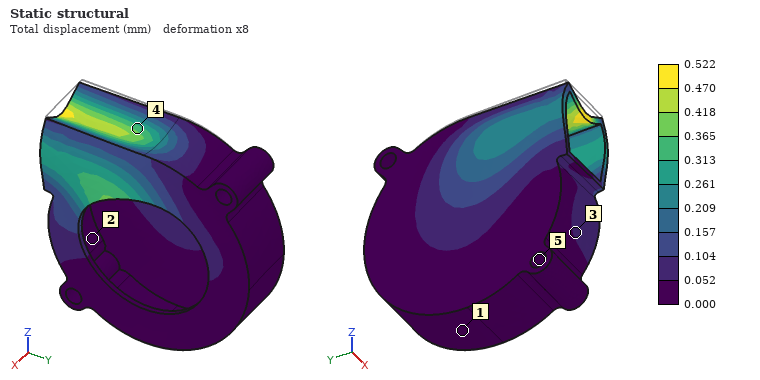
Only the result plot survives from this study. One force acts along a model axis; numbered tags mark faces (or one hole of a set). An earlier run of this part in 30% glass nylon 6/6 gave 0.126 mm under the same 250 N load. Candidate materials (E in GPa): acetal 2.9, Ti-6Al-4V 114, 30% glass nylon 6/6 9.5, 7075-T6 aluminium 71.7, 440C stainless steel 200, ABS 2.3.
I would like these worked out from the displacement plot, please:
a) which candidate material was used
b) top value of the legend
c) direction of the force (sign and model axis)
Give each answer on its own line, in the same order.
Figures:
ABS
0.522 mm
-Z
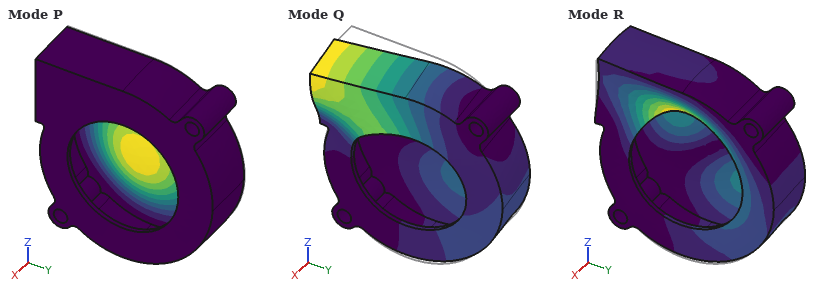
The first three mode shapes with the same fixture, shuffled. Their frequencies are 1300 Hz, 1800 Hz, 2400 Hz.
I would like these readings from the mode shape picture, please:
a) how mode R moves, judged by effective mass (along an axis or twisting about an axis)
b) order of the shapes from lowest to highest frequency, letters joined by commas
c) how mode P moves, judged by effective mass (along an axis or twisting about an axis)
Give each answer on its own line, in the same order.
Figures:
along X
P, Q, R
along X
